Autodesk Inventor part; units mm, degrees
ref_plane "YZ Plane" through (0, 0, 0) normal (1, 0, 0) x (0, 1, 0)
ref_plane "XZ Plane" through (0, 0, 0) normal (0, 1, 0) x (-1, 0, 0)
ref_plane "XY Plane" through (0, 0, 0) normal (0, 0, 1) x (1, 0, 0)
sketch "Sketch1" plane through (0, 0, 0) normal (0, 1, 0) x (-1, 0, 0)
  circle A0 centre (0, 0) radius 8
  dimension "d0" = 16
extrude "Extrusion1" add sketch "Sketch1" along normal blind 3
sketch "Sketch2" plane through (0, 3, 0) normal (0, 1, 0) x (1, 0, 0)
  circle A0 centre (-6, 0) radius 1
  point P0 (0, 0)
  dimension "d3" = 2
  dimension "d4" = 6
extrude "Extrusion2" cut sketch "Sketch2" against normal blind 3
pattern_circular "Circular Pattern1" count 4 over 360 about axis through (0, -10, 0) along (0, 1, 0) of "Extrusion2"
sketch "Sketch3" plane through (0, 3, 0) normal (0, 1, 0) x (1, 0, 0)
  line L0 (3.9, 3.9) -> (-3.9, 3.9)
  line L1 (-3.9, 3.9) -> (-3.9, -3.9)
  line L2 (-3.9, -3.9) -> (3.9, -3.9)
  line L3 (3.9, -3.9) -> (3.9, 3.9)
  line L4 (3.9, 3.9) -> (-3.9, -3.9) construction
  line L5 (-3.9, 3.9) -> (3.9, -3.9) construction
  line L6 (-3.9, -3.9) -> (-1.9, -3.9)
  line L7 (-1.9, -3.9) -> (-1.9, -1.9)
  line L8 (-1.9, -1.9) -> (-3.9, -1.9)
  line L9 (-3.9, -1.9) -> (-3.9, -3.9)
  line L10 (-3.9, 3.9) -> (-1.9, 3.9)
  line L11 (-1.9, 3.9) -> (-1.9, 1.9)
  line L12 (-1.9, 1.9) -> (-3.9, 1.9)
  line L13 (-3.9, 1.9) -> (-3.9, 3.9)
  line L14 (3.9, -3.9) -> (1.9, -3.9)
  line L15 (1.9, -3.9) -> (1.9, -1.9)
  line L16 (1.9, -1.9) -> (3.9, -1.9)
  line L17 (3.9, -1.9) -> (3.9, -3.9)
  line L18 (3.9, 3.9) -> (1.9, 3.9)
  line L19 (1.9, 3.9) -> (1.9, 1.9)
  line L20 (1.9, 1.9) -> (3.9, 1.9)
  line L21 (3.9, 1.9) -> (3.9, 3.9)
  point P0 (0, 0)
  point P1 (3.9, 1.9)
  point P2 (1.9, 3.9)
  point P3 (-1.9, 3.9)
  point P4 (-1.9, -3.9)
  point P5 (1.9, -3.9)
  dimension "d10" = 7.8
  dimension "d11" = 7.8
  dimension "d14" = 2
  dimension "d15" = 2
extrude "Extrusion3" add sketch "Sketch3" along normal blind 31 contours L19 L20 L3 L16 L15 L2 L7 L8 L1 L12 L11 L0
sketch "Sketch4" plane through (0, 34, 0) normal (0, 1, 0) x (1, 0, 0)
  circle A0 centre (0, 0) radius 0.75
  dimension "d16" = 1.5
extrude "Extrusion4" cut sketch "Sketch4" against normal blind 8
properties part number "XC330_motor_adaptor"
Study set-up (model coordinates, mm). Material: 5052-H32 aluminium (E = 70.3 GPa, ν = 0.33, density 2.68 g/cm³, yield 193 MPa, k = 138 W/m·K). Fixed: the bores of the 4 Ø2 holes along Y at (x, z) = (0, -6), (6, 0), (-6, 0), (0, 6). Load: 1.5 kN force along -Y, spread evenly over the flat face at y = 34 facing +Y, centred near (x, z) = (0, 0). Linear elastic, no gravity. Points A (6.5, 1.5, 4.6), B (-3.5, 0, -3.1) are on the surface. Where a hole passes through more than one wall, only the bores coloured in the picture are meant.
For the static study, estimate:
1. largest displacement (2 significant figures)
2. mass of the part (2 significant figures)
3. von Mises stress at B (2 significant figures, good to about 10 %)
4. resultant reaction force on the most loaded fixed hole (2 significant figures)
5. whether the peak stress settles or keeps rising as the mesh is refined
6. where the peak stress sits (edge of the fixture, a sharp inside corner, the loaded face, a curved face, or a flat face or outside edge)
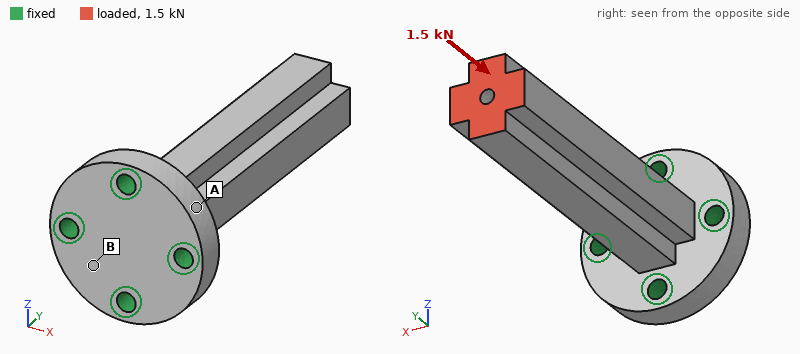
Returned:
18 µm
5.2 g
20 MPa
390 N
keeps rising
edge of the fixture
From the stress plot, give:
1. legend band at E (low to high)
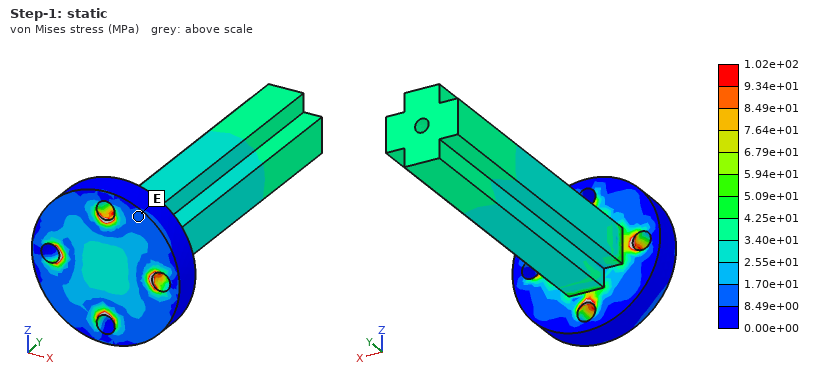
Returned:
8.49e+00 to 1.70e+01 MPa
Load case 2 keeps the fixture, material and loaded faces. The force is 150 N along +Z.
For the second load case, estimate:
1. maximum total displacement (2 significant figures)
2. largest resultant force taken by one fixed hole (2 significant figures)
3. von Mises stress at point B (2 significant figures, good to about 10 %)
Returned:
0.16 mm
440 N
20 MPa
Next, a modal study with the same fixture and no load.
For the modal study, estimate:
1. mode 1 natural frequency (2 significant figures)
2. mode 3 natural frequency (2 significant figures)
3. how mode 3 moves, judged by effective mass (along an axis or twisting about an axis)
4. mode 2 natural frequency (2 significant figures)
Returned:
5000 Hz
21 kHz
twisting about Y
5000 Hz
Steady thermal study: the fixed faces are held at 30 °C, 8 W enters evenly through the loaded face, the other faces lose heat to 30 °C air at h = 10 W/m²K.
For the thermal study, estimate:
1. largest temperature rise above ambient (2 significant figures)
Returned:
43 K
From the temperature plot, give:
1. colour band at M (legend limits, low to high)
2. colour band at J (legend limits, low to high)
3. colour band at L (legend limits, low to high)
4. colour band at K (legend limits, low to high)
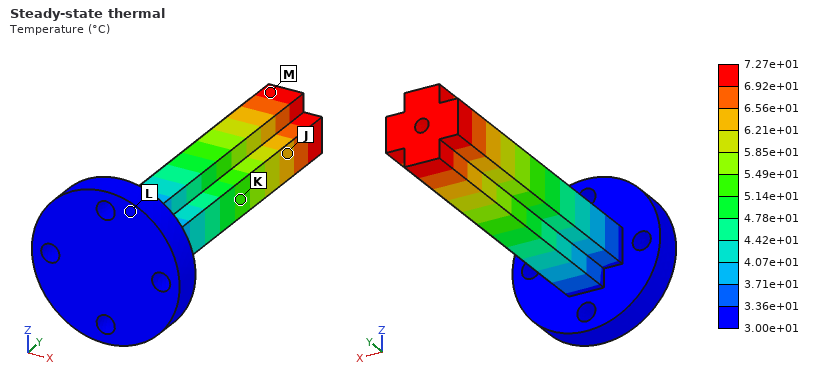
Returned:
6.92e+01 to 7.27e+01 °C
6.21e+01 to 6.56e+01 °C
3.00e+01 to 3.36e+01 °C
5.14e+01 to 5.49e+01 °C
